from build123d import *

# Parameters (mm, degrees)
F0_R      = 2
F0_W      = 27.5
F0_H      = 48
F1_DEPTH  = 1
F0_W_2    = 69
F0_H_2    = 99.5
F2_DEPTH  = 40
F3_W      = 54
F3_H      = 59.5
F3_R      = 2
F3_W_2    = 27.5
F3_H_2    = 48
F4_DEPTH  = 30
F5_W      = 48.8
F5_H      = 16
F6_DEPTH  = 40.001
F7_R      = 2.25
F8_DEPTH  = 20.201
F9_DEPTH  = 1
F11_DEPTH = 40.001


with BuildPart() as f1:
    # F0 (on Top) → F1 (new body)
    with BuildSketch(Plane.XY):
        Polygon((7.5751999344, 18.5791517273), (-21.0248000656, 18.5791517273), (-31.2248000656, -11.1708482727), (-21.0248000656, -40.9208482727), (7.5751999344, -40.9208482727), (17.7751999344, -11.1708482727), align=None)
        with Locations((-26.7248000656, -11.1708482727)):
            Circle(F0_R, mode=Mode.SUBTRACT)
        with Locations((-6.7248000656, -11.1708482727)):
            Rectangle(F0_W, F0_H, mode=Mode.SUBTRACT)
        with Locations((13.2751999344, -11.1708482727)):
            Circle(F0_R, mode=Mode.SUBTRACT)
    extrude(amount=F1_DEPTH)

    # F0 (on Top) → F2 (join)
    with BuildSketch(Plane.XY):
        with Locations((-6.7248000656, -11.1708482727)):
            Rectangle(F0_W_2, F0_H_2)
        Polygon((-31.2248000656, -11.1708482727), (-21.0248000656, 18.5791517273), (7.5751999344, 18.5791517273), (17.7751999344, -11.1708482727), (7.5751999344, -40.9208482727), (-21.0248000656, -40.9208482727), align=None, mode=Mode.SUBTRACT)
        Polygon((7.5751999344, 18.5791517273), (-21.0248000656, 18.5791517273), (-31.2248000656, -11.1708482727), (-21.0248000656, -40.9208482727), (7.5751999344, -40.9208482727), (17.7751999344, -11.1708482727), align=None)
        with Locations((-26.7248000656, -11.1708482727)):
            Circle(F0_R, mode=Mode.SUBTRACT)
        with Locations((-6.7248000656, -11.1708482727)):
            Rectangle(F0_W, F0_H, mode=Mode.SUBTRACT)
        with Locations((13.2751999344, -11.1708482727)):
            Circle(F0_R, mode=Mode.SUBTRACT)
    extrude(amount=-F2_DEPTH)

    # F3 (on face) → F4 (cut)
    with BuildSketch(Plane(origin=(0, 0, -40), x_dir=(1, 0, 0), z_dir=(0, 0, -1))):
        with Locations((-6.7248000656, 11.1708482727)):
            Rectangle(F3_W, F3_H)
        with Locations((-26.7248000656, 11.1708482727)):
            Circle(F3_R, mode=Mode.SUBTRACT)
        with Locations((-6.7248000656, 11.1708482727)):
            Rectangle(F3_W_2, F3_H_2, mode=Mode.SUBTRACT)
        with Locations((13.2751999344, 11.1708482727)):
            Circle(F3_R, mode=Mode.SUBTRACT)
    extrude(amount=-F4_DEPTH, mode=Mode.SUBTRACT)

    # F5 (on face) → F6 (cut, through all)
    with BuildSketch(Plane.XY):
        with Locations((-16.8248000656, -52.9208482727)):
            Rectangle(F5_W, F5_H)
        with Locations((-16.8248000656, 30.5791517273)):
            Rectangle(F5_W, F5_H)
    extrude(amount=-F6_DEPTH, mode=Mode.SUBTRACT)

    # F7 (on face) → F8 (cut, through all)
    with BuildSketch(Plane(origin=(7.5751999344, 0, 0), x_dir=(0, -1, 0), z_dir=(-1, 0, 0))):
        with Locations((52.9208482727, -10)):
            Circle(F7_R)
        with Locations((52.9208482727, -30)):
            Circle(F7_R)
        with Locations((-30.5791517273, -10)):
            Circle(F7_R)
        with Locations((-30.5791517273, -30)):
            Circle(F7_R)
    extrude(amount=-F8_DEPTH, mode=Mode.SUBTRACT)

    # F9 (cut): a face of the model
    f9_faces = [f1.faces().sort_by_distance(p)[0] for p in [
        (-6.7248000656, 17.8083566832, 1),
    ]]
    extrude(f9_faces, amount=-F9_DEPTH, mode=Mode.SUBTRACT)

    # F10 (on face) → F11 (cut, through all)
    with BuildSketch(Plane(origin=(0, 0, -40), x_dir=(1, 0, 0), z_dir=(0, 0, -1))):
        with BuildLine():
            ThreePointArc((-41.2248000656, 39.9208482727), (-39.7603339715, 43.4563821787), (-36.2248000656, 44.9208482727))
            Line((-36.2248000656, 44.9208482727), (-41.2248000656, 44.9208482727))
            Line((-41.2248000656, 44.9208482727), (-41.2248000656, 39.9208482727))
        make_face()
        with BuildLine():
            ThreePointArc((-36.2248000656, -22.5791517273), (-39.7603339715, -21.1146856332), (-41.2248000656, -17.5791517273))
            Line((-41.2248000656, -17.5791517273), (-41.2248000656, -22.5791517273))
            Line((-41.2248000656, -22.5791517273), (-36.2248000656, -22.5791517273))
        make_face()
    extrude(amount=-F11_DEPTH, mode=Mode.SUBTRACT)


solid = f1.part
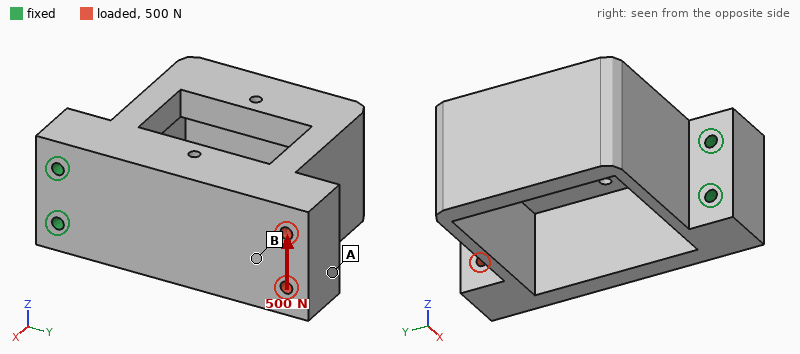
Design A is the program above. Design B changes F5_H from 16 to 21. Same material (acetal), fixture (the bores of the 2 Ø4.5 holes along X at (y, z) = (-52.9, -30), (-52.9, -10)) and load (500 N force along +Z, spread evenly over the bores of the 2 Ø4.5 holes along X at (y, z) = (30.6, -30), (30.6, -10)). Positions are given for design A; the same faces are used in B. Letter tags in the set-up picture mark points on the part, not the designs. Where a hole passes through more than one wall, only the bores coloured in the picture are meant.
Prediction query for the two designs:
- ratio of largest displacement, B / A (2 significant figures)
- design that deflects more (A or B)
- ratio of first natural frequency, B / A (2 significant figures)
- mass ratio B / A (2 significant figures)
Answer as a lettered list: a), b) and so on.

a) 1.2
b) B
c) 0.96
d) 0.91
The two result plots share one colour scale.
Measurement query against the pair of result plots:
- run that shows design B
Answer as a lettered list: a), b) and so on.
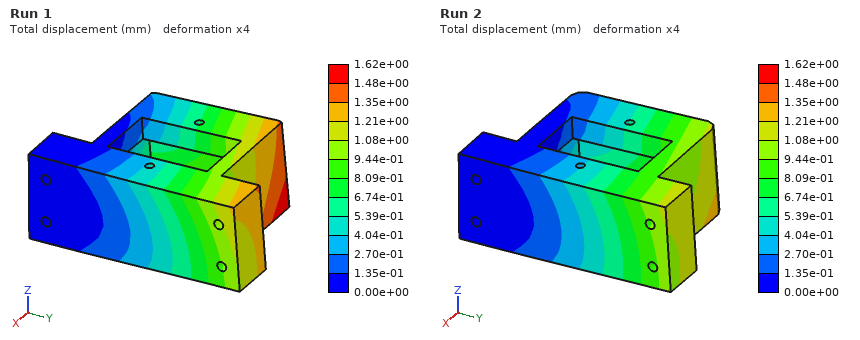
a) Run 1
